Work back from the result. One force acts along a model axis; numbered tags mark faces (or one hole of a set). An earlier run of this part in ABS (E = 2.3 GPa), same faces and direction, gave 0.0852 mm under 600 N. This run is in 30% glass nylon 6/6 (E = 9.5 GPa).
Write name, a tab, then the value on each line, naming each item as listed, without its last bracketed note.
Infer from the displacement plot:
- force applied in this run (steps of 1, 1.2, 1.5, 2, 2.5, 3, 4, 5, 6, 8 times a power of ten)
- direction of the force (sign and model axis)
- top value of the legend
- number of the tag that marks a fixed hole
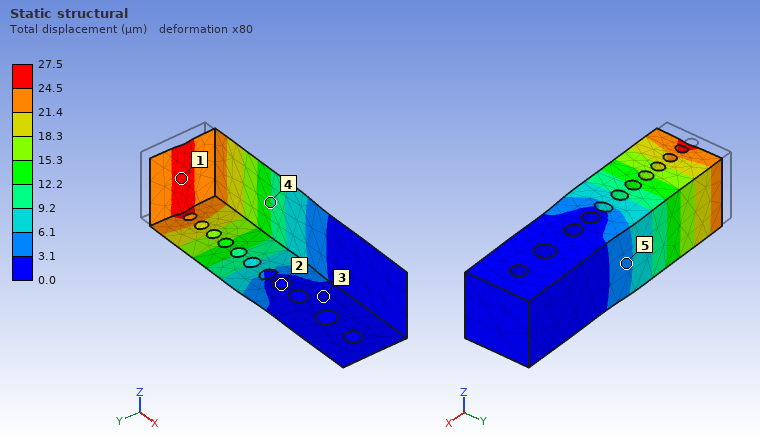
force applied in this run	800 N
direction of the force	+X
top value of the legend	27.5 µm
number of the tag that marks a fixed hole	2
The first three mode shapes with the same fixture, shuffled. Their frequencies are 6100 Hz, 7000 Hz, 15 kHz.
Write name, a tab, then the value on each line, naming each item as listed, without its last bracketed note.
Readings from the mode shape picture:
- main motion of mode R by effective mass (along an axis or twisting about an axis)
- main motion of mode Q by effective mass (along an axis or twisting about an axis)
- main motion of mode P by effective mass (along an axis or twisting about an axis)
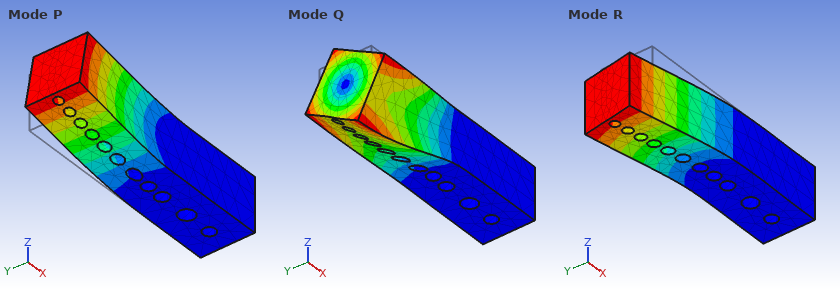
main motion of mode R by effective mass	along Y
main motion of mode Q by effective mass	twisting about X
main motion of mode P by effective mass	along Z
